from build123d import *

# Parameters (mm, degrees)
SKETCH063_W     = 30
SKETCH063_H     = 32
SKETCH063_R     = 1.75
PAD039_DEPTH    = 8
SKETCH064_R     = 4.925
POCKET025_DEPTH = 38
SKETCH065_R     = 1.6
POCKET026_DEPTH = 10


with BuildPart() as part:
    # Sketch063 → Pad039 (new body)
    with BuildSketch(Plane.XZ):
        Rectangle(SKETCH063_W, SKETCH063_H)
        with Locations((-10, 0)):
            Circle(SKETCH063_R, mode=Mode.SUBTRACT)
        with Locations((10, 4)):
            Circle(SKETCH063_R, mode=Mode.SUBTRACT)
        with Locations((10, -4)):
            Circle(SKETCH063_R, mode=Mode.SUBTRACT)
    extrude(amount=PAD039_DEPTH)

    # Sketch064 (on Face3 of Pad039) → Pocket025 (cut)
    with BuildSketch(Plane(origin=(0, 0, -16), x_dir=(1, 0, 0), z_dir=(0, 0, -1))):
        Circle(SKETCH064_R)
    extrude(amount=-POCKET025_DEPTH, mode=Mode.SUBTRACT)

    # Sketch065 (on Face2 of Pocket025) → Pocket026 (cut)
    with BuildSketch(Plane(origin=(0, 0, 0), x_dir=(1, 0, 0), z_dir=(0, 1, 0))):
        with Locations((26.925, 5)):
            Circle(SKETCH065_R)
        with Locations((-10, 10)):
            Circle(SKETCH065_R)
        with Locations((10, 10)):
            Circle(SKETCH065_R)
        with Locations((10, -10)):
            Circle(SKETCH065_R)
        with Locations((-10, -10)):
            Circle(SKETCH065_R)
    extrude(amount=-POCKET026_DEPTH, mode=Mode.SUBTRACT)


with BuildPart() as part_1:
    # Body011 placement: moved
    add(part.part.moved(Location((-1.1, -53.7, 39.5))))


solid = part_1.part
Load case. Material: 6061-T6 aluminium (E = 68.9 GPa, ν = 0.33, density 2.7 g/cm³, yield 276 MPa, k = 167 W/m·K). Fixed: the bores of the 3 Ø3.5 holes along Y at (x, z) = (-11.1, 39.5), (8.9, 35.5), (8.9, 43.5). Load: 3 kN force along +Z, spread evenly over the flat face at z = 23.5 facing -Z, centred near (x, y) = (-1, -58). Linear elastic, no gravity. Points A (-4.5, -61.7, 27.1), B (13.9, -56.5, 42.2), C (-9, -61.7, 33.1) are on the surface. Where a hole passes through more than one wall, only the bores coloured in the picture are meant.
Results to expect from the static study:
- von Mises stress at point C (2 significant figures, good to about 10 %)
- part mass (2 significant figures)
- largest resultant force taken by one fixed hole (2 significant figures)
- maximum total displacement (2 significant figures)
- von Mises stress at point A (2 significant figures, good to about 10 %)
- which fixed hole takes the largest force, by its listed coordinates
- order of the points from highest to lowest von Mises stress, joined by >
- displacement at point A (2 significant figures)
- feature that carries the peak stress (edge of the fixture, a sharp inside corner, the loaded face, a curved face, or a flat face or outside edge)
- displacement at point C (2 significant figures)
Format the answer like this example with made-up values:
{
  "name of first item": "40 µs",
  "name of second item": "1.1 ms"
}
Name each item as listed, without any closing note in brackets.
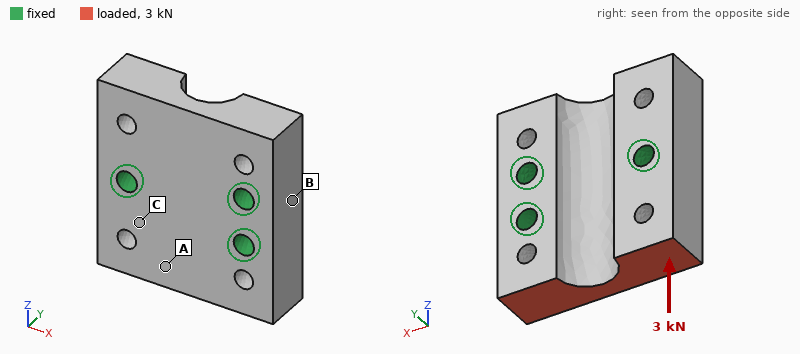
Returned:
{
  "von Mises stress at point C": "22 MPa",
  "part mass": "16 g",
  "largest resultant force taken by one fixed hole": "1.5 kN",
  "maximum total displacement": "4.9 µm",
  "von Mises stress at point A": "14 MPa",
  "which fixed hole takes the largest force, by its listed coordinates": "(-11.1, 39.5)",
  "order of the points from highest to lowest von Mises stress, joined by >": "C > A > B",
  "displacement at point A": "3.4 µm",
  "feature that carries the peak stress": "a curved face",
  "displacement at point C": "1.8 µm"
}
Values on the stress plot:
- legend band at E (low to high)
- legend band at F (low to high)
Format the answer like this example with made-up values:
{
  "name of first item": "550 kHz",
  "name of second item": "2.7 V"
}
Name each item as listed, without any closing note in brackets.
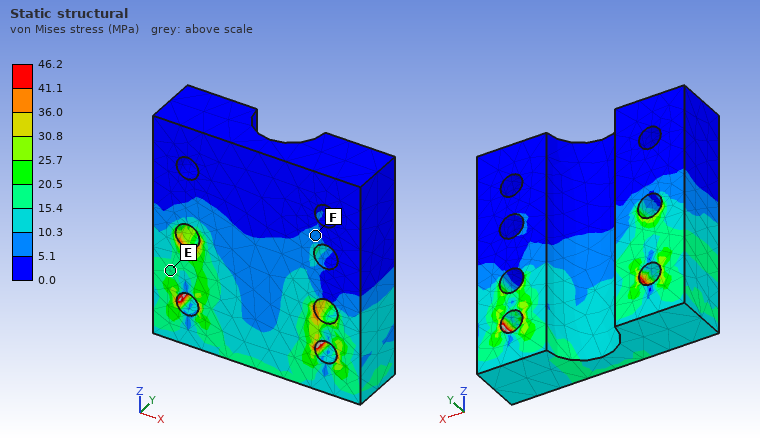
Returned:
{
  "legend band at E": "15.4 to 20.5 MPa",
  "legend band at F": "5.1 to 10.3 MPa"
}
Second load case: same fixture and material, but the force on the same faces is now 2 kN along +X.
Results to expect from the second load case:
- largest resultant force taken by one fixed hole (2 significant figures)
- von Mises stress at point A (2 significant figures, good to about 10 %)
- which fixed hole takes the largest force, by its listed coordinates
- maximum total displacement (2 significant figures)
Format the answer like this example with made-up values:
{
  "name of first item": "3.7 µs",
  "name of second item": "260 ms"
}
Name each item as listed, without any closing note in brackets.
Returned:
{
  "largest resultant force taken by one fixed hole": "1.6 kN",
  "von Mises stress at point A": "27 MPa",
  "which fixed hole takes the largest force, by its listed coordinates": "(8.9, 35.5)",
  "maximum total displacement": "17 µm"
}
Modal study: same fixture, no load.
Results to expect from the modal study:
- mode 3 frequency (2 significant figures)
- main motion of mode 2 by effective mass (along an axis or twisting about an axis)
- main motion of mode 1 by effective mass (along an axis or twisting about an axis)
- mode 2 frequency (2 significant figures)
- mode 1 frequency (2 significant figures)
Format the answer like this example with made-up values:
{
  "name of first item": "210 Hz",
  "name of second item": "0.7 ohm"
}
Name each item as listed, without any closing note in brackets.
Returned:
{
  "mode 3 frequency": "33 kHz",
  "main motion of mode 2 by effective mass": "along Y",
  "main motion of mode 1 by effective mass": "twisting about X",
  "mode 2 frequency": "25 kHz",
  "mode 1 frequency": "22 kHz"
}
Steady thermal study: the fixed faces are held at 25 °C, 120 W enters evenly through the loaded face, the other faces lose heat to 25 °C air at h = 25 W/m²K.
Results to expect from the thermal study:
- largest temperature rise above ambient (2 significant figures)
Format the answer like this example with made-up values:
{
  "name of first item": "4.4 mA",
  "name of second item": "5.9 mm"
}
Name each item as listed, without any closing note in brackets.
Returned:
{
  "largest temperature rise above ambient": "60 K"
}
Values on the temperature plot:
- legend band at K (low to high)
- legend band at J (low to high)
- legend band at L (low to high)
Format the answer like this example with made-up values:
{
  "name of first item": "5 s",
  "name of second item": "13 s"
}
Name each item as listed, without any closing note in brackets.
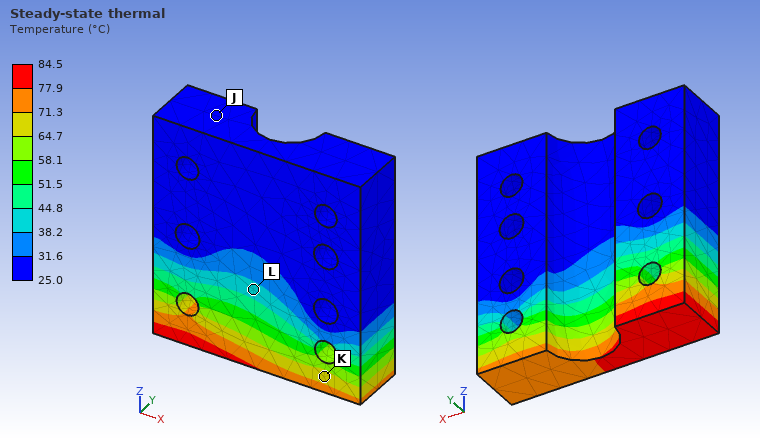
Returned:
{
  "legend band at K": "64.7 to 71.3 °C",
  "legend band at J": "25.0 to 31.6 °C",
  "legend band at L": "38.2 to 44.8 °C"
}
